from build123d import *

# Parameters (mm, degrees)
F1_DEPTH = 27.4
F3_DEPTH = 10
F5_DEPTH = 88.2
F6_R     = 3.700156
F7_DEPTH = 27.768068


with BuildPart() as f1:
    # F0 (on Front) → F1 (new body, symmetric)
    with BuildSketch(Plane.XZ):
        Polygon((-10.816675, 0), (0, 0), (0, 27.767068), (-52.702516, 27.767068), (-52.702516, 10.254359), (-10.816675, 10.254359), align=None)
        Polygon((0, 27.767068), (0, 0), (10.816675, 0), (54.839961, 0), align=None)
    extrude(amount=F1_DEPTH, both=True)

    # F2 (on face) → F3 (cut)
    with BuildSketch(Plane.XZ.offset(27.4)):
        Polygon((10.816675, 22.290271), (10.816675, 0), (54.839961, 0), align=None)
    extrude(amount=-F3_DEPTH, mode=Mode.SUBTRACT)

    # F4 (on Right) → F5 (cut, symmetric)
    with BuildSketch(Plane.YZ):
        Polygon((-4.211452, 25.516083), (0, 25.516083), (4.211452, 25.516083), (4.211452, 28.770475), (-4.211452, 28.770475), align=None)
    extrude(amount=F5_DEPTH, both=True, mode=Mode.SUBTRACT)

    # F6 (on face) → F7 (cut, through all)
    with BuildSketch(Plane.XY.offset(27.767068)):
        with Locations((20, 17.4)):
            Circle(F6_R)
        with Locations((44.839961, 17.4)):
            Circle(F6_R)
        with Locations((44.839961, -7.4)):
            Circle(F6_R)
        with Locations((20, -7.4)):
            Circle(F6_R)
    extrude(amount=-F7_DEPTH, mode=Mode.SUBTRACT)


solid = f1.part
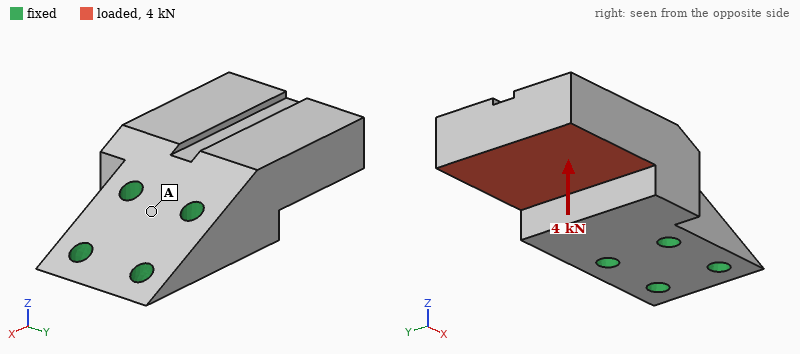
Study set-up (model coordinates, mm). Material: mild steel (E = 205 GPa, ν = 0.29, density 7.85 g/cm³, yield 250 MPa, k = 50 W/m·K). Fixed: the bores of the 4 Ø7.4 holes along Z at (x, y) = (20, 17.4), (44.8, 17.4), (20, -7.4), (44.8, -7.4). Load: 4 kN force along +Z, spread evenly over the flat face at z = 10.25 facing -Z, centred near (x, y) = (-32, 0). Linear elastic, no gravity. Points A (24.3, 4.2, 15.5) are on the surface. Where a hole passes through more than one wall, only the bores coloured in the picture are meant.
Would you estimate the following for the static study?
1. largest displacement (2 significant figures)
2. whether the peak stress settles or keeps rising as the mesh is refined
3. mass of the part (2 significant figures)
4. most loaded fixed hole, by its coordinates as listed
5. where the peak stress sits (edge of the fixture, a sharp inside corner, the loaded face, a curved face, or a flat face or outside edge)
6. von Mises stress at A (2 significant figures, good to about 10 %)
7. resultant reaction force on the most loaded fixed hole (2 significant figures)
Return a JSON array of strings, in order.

["51 µm", "keeps rising", "710 g", "(20, -7.4)", "edge of the fixture", "23 MPa", "2.7 kN"]
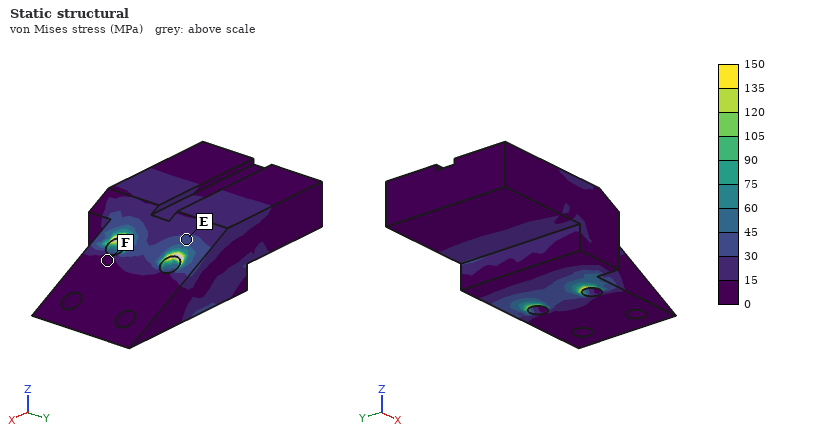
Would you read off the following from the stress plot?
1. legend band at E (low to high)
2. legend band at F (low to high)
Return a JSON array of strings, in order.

["30 to 45 MPa", "0 to 15 MPa"]
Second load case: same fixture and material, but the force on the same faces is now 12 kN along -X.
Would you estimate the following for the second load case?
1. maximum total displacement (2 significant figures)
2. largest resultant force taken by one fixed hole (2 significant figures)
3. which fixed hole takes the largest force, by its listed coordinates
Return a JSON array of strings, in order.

["21 µm", "7.7 kN", "(20, -7.4)"]
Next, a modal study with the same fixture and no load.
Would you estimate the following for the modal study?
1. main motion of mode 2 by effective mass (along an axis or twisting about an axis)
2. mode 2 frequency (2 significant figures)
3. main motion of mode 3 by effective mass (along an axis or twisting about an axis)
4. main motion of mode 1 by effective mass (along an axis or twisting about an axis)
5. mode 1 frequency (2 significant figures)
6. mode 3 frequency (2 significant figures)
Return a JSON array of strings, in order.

["along Y", "5300 Hz", "twisting about X", "along Z", "3000 Hz", "7100 Hz"]
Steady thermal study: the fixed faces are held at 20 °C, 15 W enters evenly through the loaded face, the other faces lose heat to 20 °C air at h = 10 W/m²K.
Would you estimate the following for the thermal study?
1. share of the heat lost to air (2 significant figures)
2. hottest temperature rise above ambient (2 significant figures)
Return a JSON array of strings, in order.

["6.0 %", "15 K"]
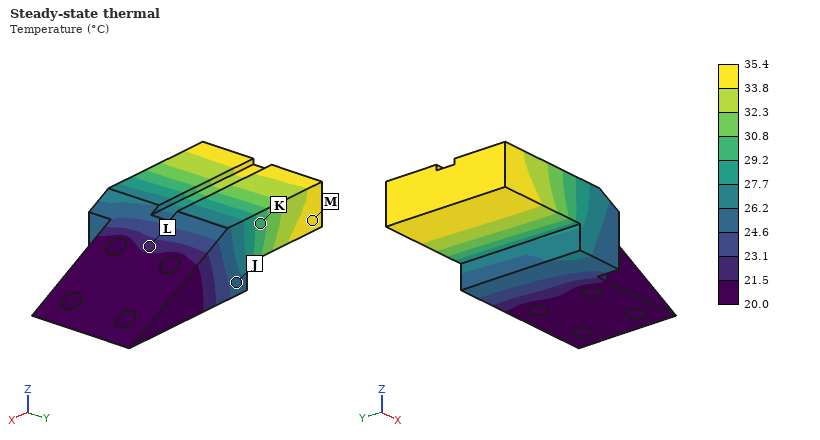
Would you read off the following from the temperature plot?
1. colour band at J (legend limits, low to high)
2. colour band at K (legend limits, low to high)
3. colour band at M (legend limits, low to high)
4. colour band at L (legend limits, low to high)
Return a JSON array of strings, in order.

["24.6 to 26.2 °C", "29.2 to 30.8 °C", "33.8 to 35.4 °C", "21.5 to 23.1 °C"]
